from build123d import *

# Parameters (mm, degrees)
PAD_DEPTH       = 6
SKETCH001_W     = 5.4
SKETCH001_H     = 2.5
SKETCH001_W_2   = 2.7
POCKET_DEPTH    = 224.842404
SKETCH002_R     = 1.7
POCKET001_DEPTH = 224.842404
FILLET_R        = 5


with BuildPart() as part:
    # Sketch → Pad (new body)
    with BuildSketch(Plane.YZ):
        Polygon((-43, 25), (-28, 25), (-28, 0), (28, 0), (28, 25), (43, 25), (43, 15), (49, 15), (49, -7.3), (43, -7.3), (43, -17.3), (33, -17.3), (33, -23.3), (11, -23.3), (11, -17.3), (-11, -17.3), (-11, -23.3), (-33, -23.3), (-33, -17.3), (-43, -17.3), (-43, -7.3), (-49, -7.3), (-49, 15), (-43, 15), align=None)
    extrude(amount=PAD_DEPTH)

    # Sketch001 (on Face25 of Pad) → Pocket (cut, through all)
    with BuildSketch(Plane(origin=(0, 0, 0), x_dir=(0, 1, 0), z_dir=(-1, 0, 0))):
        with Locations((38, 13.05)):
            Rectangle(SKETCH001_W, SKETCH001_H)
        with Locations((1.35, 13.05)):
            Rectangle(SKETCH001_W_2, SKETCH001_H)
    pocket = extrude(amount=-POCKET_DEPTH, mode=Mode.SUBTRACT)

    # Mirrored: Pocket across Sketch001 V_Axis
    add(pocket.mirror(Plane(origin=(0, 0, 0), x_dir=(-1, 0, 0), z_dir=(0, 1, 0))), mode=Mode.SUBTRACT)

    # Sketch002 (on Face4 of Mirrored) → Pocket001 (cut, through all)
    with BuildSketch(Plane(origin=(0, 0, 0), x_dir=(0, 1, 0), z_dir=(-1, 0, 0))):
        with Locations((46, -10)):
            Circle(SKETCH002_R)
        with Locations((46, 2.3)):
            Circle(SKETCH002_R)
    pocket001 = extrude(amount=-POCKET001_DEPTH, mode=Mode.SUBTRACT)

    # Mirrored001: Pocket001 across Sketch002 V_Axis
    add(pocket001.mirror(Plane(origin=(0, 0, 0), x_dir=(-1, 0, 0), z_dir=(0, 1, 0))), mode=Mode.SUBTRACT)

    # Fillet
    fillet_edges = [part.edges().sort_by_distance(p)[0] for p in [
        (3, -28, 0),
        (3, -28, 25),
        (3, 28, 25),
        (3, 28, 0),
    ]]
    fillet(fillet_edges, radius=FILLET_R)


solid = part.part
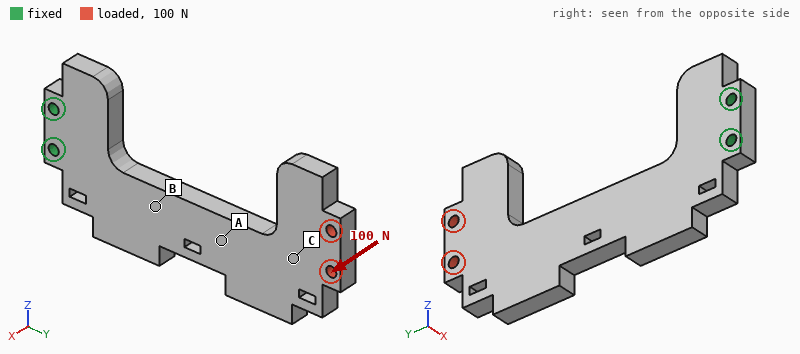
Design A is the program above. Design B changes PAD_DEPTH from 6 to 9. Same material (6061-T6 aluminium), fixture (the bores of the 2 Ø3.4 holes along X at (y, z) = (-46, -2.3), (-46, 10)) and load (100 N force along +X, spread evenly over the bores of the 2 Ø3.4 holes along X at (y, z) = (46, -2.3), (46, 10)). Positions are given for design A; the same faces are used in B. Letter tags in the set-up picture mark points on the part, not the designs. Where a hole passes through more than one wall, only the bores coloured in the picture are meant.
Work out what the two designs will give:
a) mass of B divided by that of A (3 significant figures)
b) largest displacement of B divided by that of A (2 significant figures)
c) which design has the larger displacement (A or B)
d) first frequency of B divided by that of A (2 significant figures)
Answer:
1.50
0.31
A
1.5
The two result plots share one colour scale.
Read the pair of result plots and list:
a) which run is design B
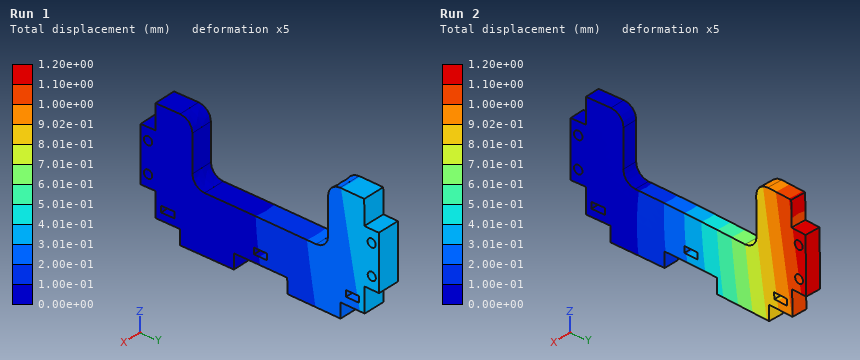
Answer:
Run 1
